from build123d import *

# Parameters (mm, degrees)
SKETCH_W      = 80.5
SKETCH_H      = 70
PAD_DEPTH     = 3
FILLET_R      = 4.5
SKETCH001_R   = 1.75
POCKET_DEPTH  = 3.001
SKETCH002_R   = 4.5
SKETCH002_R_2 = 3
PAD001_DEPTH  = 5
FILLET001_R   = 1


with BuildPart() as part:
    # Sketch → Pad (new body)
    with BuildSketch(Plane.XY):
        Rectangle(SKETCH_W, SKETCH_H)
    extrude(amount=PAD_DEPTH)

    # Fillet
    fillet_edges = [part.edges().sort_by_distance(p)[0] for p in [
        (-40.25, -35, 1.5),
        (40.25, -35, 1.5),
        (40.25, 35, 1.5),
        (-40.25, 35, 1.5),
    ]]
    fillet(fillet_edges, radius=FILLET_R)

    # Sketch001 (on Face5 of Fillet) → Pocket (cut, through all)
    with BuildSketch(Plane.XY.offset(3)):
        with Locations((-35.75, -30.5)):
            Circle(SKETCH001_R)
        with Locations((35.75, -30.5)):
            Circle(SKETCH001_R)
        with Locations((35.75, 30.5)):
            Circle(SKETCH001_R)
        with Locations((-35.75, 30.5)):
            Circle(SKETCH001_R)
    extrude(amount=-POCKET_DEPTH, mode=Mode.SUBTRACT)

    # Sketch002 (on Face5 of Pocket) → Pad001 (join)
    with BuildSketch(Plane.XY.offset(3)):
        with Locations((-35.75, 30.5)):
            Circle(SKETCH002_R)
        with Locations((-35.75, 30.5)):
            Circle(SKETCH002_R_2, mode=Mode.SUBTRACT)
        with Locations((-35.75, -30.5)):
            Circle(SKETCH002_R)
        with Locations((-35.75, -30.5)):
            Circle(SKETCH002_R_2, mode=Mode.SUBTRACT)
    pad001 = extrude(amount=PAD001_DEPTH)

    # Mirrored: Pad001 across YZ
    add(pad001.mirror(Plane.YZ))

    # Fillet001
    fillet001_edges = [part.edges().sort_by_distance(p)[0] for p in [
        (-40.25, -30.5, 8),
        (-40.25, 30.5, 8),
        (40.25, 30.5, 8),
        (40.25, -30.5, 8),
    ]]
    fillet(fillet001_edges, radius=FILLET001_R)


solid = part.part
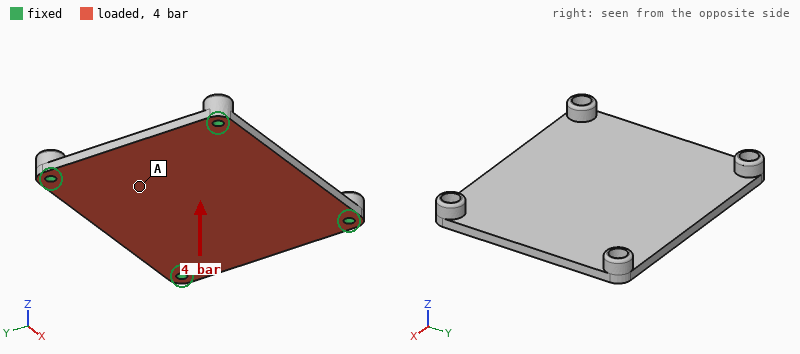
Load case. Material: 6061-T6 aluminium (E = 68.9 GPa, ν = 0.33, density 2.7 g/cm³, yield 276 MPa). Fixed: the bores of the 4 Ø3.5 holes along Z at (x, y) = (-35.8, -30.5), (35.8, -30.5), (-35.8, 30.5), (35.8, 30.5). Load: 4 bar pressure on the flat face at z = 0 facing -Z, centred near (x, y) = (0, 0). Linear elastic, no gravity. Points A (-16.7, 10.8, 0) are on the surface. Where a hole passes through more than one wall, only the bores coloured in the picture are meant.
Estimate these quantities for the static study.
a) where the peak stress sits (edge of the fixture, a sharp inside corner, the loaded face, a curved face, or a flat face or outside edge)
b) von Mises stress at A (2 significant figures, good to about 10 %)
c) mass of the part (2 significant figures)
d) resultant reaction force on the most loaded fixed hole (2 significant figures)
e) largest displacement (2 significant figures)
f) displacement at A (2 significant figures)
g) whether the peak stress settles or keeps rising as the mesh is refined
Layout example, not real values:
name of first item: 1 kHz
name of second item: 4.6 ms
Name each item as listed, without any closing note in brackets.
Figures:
where the peak stress sits: edge of the fixture
von Mises stress at A: 46 MPa
mass of the part: 47 g
resultant reaction force on the most loaded fixed hole: 560 N
largest displacement: 0.35 mm
displacement at A: 0.26 mm
whether the peak stress settles or keeps rising as the mesh is refined: keeps rising
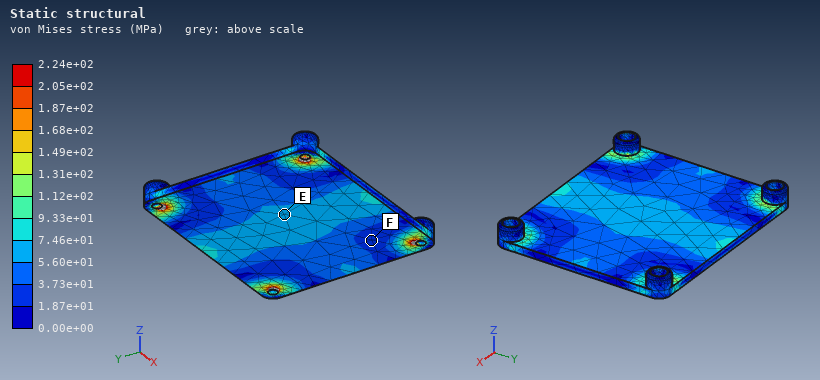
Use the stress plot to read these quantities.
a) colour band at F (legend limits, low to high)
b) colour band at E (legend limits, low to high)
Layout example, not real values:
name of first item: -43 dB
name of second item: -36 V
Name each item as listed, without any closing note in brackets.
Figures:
colour band at F: 1.87e+01 to 3.73e+01 MPa
colour band at E: 5.60e+01 to 7.46e+01 MPa
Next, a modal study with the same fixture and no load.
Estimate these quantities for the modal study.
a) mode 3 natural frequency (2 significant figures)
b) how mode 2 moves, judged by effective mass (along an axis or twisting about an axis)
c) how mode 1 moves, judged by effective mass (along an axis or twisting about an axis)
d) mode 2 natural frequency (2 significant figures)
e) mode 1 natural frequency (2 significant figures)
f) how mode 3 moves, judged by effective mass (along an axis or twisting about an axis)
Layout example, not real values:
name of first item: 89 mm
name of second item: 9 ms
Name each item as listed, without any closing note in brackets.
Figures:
mode 3 natural frequency: 4400 Hz
how mode 2 moves, judged by effective mass: twisting about X
how mode 1 moves, judged by effective mass: along Z
mode 2 natural frequency: 3700 Hz
mode 1 natural frequency: 2300 Hz
how mode 3 moves, judged by effective mass: twisting about Y
